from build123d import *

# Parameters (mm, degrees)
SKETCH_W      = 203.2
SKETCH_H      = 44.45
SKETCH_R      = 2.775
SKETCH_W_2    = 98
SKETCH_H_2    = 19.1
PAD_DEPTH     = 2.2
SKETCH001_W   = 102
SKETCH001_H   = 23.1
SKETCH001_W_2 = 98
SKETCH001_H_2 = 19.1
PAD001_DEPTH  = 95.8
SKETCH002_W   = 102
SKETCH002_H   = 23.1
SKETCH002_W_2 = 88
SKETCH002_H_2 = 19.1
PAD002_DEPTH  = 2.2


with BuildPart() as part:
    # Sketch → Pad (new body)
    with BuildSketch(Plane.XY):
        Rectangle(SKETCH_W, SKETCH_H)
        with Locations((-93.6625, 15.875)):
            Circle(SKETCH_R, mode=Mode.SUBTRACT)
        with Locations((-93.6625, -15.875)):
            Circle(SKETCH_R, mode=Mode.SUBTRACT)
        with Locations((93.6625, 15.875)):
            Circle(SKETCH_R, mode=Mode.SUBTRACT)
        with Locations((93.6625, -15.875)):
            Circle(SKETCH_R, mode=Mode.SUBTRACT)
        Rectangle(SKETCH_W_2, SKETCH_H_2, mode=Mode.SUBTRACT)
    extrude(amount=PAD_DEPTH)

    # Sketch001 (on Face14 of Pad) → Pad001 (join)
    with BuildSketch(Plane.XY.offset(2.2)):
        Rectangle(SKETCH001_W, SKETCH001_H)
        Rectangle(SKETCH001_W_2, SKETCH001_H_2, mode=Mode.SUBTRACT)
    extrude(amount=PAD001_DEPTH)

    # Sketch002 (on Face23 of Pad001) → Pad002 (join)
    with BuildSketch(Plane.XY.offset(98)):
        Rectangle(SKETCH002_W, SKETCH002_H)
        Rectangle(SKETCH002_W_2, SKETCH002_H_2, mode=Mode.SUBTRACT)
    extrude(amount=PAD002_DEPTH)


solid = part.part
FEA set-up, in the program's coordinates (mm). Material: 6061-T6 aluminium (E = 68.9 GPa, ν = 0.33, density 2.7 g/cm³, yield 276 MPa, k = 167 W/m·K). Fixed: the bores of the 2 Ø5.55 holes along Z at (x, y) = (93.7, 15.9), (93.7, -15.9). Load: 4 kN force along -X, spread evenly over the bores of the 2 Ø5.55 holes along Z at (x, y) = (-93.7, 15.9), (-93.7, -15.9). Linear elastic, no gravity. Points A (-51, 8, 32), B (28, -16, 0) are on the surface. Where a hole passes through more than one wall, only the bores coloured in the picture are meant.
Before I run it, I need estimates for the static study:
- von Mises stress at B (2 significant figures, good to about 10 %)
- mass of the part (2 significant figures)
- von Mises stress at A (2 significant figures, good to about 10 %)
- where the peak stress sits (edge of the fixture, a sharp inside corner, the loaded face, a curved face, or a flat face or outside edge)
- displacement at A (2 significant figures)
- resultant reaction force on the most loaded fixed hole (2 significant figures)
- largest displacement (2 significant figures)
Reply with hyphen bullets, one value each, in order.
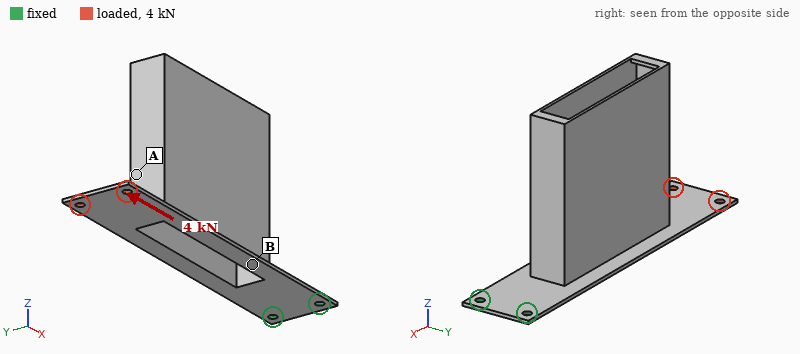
- 44 MPa
- 170 g
- 12 MPa
- the loaded face
- 0.28 mm
- 2.0 kN
- 0.59 mm
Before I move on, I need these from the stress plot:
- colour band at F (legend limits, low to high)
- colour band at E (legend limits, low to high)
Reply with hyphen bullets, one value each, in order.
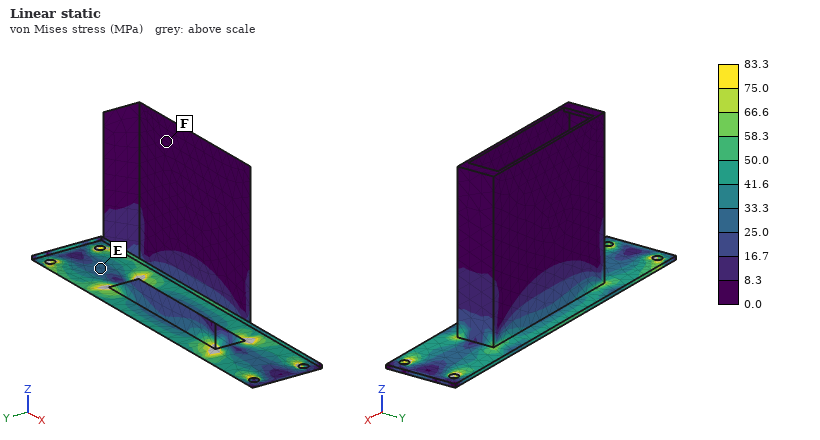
- 0.0 to 8.3 MPa
- 25.0 to 33.3 MPa
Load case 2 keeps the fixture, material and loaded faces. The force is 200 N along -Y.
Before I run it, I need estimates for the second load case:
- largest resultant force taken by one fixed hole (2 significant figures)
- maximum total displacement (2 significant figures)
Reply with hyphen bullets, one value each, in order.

- 1.1 kN
- 0.69 mm
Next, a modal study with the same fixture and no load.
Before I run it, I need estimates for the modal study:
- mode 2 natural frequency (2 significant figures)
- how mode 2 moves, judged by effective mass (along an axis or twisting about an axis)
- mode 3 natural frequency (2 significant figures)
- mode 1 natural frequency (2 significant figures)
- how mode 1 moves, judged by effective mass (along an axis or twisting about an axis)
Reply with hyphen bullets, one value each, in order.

- 93 Hz
- along Y
- 380 Hz
- 32 Hz
- along Z
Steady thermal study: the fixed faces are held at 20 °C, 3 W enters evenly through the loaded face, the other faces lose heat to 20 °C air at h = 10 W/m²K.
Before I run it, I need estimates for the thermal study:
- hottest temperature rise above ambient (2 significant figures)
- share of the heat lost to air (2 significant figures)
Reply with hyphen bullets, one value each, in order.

- 15 K
- 78 %
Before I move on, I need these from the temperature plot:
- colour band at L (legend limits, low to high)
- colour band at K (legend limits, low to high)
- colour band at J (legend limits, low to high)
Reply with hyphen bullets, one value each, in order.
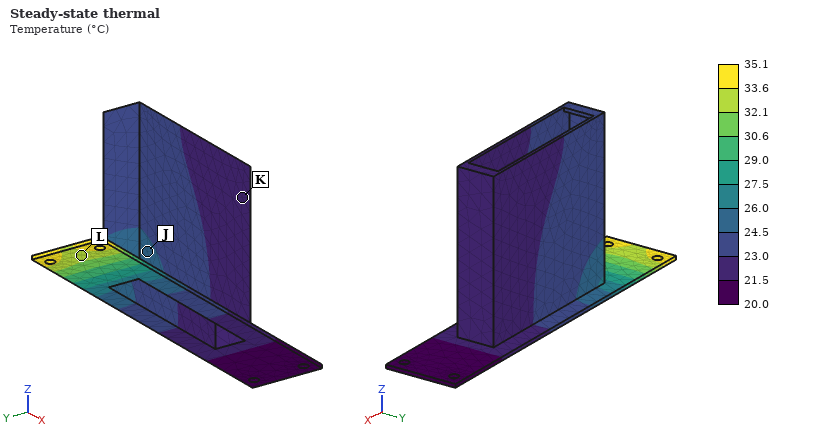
- 32.1 to 33.6 °C
- 21.5 to 23.0 °C
- 24.5 to 26.0 °C
